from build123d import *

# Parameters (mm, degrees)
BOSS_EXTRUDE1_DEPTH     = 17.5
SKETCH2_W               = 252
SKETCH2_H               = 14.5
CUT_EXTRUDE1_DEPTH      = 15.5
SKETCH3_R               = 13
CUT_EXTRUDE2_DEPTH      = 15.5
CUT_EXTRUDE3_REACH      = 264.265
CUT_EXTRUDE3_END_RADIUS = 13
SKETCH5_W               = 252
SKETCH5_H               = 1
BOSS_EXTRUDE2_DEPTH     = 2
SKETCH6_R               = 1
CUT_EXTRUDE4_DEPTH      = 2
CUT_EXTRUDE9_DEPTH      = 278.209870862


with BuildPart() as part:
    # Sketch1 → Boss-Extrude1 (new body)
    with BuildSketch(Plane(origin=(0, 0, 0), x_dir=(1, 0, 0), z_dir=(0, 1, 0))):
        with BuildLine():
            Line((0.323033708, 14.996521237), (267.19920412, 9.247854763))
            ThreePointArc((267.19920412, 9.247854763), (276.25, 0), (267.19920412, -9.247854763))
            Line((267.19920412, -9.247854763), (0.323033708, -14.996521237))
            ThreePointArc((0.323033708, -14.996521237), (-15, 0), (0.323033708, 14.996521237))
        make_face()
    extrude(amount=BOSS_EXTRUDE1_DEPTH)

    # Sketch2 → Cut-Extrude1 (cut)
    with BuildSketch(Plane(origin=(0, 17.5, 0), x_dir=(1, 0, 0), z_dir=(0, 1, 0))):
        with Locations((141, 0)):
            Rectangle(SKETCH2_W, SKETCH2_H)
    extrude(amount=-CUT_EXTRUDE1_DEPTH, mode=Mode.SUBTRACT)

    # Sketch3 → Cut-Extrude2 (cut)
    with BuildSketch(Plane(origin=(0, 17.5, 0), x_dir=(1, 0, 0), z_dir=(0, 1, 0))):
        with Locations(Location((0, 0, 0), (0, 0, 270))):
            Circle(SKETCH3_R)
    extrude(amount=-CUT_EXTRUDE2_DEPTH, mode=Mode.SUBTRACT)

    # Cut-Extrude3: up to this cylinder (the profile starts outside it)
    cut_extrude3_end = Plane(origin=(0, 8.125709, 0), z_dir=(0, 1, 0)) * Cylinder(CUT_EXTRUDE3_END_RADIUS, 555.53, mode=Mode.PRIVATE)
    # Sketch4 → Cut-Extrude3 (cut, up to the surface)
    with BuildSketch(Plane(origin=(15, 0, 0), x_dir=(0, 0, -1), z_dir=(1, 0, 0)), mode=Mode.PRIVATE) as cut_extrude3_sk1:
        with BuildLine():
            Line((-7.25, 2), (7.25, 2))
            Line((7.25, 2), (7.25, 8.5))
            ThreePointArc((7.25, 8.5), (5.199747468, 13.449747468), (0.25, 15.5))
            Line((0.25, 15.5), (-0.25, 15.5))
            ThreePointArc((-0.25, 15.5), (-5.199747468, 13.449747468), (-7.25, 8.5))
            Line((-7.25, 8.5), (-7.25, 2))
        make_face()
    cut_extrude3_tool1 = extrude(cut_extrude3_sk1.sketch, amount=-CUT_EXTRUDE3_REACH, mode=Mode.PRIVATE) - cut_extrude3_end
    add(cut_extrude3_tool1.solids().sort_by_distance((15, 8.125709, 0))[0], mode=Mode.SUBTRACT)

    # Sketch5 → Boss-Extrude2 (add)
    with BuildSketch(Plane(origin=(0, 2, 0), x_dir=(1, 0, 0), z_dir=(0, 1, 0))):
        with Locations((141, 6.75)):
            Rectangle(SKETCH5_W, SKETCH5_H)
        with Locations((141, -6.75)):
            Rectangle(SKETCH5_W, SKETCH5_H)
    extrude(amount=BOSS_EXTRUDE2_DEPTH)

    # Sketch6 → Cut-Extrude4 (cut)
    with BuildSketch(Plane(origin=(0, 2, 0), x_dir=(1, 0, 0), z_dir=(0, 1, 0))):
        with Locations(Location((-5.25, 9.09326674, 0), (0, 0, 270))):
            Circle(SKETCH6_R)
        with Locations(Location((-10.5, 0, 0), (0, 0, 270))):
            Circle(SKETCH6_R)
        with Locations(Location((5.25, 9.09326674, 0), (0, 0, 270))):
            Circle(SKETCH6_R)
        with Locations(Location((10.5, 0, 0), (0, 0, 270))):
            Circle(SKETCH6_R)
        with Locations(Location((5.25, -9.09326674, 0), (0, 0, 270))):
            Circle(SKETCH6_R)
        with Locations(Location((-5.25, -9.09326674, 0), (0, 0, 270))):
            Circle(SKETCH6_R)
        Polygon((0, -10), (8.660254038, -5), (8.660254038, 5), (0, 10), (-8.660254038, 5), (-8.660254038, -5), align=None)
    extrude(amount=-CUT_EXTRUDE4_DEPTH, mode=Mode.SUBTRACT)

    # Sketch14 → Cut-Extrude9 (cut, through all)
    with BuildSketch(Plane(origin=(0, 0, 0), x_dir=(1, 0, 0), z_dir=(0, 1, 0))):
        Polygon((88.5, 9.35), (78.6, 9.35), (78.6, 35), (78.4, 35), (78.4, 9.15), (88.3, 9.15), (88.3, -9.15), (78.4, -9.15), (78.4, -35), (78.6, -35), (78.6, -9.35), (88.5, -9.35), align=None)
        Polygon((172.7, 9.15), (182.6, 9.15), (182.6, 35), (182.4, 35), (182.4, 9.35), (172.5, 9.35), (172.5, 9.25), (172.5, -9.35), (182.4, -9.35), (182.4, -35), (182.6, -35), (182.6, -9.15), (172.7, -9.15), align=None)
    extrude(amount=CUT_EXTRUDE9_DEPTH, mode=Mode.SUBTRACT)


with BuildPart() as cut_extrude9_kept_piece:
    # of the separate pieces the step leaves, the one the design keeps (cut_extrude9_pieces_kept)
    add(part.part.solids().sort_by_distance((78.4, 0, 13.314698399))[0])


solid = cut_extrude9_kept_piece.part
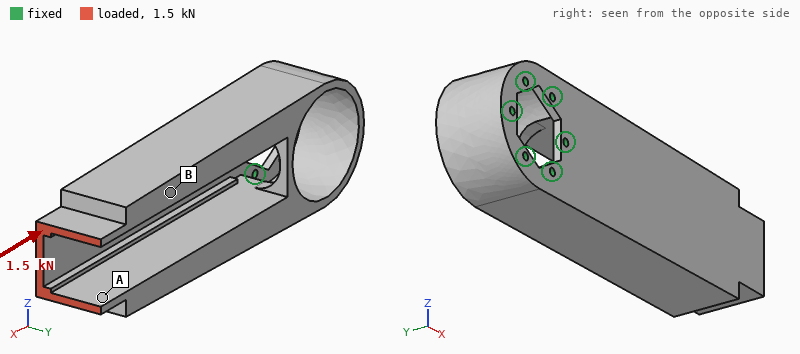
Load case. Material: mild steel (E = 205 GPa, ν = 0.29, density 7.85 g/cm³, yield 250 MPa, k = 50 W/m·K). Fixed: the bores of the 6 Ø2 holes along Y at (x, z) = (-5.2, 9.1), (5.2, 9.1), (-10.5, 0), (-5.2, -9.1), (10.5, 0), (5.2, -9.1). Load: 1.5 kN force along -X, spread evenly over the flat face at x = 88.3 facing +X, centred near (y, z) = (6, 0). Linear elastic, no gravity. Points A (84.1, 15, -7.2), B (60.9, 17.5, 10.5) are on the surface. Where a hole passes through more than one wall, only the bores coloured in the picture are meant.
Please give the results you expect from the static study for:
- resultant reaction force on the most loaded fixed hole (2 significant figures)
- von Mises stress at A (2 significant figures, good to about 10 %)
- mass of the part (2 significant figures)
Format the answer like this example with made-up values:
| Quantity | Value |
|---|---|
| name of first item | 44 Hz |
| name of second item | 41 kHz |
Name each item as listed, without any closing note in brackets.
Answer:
| Quantity | Value |
|---|---|
| resultant reaction force on the most loaded fixed hole | 440 N |
| von Mises stress at A | 14 MPa |
| mass of the part | 180 g |
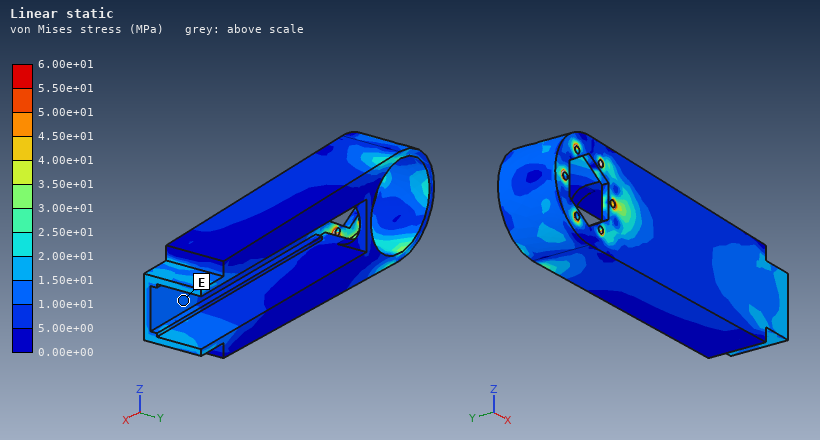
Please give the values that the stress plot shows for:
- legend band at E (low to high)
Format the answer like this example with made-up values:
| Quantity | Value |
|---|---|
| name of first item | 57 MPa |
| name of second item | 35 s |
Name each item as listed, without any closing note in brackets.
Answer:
| Quantity | Value |
|---|---|
| legend band at E | 1.00e+01 to 1.50e+01 MPa |
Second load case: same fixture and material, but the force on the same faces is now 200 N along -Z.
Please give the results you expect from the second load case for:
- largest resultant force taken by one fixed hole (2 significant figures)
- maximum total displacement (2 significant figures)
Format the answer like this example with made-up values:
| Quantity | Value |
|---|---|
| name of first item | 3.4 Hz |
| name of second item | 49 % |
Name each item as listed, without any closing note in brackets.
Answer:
| Quantity | Value |
|---|---|
| largest resultant force taken by one fixed hole | 490 N |
| maximum total displacement | 41 µm |
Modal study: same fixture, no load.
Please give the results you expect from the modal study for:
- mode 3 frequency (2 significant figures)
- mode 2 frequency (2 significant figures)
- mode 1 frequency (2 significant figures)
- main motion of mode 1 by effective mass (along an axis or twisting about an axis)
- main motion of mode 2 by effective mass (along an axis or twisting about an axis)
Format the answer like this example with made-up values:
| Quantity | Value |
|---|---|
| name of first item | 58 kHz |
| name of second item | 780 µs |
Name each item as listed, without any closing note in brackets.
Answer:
| Quantity | Value |
|---|---|
| mode 3 frequency | 3000 Hz |
| mode 2 frequency | 1900 Hz |
| mode 1 frequency | 1100 Hz |
| main motion of mode 1 by effective mass | along Y |
| main motion of mode 2 by effective mass | along Z |
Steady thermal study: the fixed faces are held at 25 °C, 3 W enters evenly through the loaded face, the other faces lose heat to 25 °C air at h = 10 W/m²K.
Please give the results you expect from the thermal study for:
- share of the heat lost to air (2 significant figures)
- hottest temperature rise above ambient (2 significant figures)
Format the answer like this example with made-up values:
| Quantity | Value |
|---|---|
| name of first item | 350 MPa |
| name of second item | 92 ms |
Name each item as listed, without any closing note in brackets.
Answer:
| Quantity | Value |
|---|---|
| share of the heat lost to air | 32 % |
| hottest temperature rise above ambient | 22 K |
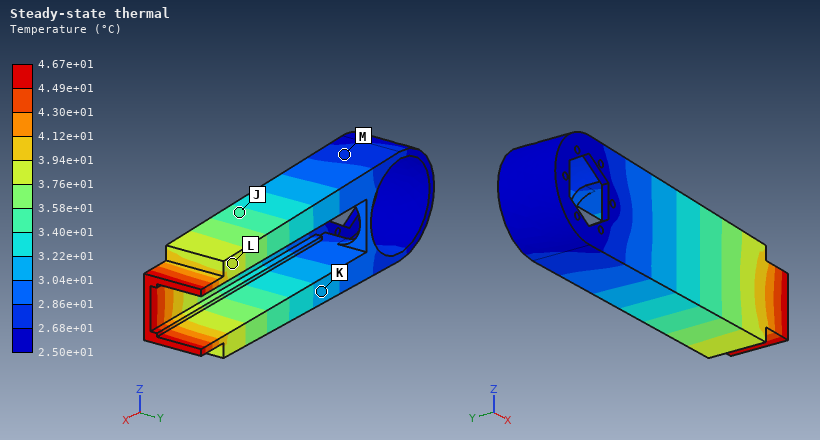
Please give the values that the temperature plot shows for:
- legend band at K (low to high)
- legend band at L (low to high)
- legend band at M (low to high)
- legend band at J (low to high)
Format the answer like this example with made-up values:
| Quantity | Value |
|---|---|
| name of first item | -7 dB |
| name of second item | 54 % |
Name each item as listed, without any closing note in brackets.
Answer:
| Quantity | Value |
|---|---|
| legend band at K | 3.04e+01 to 3.22e+01 °C |
| legend band at L | 3.76e+01 to 3.94e+01 °C |
| legend band at M | 2.68e+01 to 2.86e+01 °C |
| legend band at J | 3.40e+01 to 3.58e+01 °C |
